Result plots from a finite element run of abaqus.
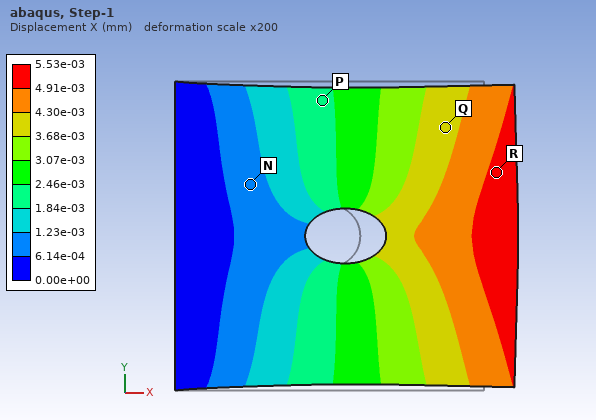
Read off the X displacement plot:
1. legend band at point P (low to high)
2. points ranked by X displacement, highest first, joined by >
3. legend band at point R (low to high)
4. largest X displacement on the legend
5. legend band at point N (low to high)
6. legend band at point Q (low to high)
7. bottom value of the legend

1.84e-03 to 2.46e-03 mm
R > Q > P > N
4.91e-03 to 5.53e-03 mm
5.53e-03 mm
6.14e-04 to 1.23e-03 mm
3.68e-03 to 4.30e-03 mm
0.00e+00 mm
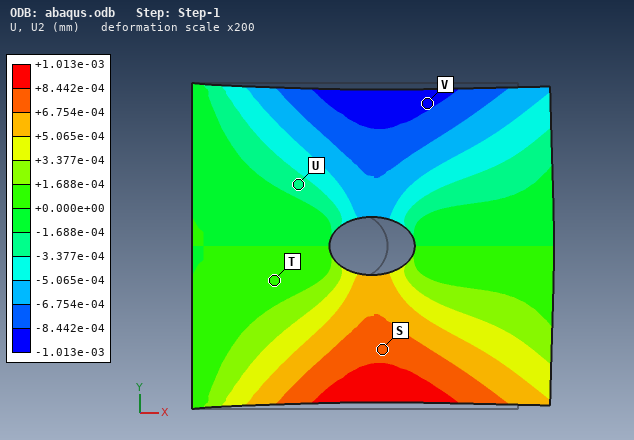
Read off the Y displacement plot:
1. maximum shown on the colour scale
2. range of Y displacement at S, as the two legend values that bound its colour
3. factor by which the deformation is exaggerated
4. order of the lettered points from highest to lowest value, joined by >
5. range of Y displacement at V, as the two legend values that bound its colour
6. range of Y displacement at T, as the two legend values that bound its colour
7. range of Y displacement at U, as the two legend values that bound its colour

+1.013e-03 mm
+6.754e-04 to +8.442e-04 mm
200
S > T > U > V
-1.013e-03 to -8.442e-04 mm
+0.000e+00 to +1.688e-04 mm
-3.377e-04 to -1.688e-04 mm
